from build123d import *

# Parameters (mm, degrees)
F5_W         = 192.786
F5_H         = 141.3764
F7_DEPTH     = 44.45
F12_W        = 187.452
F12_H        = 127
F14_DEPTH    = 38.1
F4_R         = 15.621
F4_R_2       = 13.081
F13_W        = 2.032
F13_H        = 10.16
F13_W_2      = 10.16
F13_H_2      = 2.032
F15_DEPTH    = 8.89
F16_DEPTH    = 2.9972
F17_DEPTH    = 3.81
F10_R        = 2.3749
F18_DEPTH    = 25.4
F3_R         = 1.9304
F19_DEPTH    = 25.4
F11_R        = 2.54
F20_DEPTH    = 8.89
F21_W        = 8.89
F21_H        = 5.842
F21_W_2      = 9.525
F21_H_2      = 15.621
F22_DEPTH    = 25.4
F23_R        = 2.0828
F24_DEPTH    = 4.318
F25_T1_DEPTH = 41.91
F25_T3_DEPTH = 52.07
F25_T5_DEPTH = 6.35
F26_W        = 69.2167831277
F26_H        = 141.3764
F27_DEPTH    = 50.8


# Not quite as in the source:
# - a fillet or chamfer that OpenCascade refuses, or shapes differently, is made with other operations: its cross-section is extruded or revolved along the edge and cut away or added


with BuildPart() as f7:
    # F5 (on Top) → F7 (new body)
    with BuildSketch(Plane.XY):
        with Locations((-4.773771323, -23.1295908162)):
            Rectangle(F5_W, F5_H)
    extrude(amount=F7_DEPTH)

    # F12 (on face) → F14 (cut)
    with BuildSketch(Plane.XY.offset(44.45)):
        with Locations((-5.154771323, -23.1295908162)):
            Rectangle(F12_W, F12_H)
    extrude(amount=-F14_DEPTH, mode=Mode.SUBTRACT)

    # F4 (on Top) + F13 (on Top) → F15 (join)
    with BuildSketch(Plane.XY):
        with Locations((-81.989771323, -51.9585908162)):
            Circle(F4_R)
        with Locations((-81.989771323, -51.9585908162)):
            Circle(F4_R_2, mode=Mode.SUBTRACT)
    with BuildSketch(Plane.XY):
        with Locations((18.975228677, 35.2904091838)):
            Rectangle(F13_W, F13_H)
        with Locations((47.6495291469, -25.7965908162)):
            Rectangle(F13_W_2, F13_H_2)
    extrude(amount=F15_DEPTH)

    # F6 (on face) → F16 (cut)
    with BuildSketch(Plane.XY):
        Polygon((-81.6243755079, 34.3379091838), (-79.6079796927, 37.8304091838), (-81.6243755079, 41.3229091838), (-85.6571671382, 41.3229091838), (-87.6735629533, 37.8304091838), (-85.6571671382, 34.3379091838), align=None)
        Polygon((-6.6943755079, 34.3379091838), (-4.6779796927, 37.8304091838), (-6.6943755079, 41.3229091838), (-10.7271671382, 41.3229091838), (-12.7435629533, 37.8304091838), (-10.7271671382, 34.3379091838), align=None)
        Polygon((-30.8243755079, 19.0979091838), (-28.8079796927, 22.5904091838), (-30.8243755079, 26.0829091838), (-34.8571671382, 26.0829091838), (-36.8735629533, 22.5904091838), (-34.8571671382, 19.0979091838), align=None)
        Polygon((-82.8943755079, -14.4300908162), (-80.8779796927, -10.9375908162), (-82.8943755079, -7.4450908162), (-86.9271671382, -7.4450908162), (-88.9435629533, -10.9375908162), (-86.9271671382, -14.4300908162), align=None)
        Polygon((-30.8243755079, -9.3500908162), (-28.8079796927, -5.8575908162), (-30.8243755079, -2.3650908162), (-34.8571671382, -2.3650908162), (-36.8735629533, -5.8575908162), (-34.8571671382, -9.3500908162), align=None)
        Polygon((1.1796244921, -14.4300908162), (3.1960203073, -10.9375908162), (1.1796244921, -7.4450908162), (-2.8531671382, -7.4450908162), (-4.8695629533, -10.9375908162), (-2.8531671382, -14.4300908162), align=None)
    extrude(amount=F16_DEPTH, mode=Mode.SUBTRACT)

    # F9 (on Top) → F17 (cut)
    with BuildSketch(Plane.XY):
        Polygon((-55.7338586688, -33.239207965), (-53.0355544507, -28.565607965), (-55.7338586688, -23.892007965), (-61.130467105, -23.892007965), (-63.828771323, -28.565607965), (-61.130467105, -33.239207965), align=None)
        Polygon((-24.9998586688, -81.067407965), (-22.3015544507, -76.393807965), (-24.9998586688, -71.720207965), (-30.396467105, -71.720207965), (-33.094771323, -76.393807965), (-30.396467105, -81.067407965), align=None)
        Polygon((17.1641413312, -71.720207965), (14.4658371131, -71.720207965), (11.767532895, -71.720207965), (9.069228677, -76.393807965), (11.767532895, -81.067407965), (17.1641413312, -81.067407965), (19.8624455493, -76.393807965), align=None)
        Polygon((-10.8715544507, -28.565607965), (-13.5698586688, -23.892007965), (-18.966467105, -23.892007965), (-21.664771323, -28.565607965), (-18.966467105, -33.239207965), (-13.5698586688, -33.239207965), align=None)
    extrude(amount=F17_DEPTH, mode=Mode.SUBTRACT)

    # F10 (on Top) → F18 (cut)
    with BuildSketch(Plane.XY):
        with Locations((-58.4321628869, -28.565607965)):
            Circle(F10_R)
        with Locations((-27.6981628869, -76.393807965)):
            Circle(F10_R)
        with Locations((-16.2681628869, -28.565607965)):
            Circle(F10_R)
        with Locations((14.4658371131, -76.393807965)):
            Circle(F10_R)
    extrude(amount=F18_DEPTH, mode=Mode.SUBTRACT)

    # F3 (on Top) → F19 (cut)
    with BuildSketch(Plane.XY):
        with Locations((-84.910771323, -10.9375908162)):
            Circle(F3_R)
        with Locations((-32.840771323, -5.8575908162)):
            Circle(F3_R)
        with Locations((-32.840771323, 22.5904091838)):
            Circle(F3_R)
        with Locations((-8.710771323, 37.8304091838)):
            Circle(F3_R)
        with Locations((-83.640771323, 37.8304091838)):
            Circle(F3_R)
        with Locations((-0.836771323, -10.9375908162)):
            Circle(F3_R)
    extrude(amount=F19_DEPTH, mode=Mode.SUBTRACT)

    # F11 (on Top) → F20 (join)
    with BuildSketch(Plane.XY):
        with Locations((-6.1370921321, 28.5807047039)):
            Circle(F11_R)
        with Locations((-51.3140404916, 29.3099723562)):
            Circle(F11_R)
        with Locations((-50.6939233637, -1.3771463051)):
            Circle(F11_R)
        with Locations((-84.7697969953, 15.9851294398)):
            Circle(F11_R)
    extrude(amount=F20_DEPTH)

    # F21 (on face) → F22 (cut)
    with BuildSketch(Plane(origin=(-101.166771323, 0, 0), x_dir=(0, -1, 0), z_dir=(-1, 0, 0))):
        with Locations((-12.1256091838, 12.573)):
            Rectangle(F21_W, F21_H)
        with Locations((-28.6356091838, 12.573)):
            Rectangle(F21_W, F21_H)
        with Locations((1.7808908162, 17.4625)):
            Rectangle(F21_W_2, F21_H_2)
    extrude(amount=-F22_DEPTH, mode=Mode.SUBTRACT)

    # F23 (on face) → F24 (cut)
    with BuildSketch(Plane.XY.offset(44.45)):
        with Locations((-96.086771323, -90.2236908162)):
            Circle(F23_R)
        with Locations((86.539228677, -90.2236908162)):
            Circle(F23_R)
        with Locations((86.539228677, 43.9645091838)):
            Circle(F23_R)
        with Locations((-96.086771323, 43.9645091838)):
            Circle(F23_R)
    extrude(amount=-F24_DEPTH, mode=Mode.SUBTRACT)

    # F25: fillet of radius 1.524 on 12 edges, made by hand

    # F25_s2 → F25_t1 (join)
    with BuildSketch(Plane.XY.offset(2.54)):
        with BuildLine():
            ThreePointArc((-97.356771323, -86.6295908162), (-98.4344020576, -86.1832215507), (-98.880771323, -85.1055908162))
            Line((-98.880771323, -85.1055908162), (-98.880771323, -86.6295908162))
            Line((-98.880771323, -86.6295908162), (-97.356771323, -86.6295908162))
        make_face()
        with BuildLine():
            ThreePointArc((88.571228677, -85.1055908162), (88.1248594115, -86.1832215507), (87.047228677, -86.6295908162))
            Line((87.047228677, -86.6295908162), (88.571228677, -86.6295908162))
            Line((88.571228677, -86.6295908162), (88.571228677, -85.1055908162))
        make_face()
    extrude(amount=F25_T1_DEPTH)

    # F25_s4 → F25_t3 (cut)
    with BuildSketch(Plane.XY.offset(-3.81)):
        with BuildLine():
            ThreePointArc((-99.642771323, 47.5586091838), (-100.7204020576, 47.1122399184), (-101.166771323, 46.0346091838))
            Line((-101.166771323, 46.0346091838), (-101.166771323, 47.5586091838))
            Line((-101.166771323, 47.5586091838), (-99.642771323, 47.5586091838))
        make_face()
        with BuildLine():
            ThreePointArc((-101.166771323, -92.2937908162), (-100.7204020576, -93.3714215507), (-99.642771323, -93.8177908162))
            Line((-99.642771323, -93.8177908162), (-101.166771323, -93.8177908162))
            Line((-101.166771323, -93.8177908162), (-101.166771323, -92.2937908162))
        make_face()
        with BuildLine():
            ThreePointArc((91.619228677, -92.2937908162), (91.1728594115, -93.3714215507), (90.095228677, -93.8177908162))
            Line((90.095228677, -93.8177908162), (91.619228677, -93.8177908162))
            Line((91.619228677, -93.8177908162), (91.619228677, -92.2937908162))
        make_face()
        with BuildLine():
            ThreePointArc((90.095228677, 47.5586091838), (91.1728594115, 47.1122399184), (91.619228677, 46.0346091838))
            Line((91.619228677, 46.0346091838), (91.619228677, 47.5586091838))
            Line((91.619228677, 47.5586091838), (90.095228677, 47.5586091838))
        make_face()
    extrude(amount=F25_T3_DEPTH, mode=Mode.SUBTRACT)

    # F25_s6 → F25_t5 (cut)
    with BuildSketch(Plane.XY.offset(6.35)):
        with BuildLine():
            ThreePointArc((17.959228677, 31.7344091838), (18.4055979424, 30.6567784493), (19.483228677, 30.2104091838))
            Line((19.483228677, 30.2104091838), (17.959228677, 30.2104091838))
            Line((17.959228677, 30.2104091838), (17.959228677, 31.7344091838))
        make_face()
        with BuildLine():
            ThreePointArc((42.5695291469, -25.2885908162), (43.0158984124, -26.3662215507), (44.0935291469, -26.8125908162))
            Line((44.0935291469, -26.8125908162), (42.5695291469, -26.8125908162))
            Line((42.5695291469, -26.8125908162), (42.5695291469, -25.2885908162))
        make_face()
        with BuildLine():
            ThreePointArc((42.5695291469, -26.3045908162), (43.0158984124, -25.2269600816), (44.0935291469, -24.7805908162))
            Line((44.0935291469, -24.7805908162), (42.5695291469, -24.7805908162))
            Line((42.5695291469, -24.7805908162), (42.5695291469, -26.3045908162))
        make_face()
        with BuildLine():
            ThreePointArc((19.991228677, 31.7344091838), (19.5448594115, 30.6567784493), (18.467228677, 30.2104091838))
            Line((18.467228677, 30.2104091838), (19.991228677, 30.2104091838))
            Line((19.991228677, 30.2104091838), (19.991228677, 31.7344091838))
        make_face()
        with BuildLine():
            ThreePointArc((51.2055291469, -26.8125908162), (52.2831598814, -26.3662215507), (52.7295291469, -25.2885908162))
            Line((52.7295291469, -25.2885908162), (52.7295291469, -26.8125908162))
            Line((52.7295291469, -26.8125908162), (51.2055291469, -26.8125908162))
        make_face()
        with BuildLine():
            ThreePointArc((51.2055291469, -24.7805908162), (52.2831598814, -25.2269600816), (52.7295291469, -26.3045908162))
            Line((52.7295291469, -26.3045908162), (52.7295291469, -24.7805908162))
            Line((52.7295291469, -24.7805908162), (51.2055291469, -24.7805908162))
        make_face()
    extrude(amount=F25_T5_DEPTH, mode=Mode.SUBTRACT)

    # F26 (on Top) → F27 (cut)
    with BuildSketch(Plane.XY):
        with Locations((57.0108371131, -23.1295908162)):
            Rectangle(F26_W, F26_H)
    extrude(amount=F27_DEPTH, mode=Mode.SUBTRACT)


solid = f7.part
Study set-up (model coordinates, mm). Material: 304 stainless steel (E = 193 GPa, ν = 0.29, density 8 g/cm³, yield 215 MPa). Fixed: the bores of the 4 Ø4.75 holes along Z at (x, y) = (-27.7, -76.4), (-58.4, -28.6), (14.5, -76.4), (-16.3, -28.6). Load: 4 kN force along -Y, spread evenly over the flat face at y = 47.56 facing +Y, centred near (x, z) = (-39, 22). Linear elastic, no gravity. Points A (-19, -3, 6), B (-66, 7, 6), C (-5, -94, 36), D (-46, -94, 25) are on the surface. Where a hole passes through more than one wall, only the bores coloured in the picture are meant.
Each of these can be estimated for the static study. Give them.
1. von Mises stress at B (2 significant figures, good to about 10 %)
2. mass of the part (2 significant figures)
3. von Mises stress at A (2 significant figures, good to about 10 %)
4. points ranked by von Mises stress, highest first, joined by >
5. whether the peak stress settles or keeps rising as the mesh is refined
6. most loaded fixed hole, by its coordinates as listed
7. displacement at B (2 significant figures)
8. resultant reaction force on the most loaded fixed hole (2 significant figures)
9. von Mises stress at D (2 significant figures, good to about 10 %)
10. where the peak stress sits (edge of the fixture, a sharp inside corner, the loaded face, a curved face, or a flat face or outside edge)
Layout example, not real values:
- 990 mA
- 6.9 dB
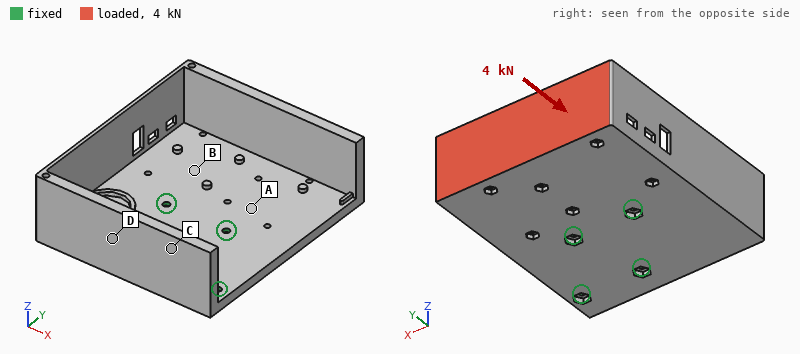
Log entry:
- 29 MPa
- 1.5 kg
- 50 MPa
- A > B > D > C
- keeps rising
- (-58.4, -28.6)
- 0.078 mm
- 2.6 kN
- 16 MPa
- edge of the fixture
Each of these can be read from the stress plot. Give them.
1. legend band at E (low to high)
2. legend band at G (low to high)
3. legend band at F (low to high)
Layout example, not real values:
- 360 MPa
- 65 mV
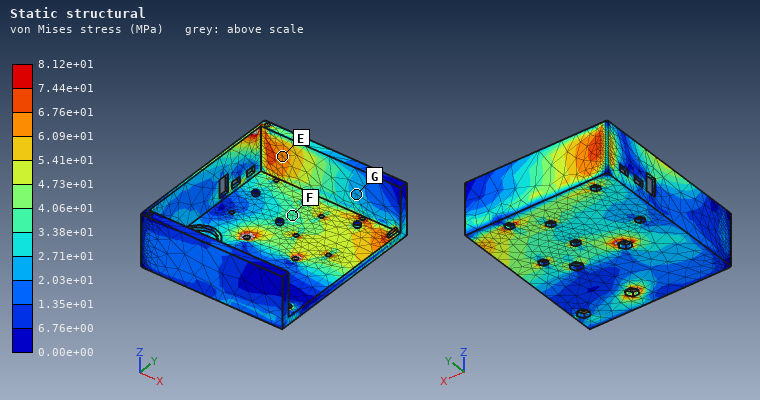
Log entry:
- 6.09e+01 to 6.76e+01 MPa
- 2.03e+01 to 2.71e+01 MPa
- 3.38e+01 to 4.06e+01 MPa
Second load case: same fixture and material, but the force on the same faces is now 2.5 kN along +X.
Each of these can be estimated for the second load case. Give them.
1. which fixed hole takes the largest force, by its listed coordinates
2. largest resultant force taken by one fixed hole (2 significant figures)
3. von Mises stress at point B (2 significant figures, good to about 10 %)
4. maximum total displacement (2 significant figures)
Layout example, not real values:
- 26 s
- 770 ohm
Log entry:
- (-58.4, -28.6)
- 3.0 kN
- 29 MPa
- 0.21 mm
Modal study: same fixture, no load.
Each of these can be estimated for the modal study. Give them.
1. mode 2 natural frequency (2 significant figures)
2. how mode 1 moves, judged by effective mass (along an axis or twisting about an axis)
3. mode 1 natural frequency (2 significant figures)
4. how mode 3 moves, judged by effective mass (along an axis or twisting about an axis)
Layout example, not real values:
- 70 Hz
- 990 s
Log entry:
- 710 Hz
- along Z
- 500 Hz
- along Z
